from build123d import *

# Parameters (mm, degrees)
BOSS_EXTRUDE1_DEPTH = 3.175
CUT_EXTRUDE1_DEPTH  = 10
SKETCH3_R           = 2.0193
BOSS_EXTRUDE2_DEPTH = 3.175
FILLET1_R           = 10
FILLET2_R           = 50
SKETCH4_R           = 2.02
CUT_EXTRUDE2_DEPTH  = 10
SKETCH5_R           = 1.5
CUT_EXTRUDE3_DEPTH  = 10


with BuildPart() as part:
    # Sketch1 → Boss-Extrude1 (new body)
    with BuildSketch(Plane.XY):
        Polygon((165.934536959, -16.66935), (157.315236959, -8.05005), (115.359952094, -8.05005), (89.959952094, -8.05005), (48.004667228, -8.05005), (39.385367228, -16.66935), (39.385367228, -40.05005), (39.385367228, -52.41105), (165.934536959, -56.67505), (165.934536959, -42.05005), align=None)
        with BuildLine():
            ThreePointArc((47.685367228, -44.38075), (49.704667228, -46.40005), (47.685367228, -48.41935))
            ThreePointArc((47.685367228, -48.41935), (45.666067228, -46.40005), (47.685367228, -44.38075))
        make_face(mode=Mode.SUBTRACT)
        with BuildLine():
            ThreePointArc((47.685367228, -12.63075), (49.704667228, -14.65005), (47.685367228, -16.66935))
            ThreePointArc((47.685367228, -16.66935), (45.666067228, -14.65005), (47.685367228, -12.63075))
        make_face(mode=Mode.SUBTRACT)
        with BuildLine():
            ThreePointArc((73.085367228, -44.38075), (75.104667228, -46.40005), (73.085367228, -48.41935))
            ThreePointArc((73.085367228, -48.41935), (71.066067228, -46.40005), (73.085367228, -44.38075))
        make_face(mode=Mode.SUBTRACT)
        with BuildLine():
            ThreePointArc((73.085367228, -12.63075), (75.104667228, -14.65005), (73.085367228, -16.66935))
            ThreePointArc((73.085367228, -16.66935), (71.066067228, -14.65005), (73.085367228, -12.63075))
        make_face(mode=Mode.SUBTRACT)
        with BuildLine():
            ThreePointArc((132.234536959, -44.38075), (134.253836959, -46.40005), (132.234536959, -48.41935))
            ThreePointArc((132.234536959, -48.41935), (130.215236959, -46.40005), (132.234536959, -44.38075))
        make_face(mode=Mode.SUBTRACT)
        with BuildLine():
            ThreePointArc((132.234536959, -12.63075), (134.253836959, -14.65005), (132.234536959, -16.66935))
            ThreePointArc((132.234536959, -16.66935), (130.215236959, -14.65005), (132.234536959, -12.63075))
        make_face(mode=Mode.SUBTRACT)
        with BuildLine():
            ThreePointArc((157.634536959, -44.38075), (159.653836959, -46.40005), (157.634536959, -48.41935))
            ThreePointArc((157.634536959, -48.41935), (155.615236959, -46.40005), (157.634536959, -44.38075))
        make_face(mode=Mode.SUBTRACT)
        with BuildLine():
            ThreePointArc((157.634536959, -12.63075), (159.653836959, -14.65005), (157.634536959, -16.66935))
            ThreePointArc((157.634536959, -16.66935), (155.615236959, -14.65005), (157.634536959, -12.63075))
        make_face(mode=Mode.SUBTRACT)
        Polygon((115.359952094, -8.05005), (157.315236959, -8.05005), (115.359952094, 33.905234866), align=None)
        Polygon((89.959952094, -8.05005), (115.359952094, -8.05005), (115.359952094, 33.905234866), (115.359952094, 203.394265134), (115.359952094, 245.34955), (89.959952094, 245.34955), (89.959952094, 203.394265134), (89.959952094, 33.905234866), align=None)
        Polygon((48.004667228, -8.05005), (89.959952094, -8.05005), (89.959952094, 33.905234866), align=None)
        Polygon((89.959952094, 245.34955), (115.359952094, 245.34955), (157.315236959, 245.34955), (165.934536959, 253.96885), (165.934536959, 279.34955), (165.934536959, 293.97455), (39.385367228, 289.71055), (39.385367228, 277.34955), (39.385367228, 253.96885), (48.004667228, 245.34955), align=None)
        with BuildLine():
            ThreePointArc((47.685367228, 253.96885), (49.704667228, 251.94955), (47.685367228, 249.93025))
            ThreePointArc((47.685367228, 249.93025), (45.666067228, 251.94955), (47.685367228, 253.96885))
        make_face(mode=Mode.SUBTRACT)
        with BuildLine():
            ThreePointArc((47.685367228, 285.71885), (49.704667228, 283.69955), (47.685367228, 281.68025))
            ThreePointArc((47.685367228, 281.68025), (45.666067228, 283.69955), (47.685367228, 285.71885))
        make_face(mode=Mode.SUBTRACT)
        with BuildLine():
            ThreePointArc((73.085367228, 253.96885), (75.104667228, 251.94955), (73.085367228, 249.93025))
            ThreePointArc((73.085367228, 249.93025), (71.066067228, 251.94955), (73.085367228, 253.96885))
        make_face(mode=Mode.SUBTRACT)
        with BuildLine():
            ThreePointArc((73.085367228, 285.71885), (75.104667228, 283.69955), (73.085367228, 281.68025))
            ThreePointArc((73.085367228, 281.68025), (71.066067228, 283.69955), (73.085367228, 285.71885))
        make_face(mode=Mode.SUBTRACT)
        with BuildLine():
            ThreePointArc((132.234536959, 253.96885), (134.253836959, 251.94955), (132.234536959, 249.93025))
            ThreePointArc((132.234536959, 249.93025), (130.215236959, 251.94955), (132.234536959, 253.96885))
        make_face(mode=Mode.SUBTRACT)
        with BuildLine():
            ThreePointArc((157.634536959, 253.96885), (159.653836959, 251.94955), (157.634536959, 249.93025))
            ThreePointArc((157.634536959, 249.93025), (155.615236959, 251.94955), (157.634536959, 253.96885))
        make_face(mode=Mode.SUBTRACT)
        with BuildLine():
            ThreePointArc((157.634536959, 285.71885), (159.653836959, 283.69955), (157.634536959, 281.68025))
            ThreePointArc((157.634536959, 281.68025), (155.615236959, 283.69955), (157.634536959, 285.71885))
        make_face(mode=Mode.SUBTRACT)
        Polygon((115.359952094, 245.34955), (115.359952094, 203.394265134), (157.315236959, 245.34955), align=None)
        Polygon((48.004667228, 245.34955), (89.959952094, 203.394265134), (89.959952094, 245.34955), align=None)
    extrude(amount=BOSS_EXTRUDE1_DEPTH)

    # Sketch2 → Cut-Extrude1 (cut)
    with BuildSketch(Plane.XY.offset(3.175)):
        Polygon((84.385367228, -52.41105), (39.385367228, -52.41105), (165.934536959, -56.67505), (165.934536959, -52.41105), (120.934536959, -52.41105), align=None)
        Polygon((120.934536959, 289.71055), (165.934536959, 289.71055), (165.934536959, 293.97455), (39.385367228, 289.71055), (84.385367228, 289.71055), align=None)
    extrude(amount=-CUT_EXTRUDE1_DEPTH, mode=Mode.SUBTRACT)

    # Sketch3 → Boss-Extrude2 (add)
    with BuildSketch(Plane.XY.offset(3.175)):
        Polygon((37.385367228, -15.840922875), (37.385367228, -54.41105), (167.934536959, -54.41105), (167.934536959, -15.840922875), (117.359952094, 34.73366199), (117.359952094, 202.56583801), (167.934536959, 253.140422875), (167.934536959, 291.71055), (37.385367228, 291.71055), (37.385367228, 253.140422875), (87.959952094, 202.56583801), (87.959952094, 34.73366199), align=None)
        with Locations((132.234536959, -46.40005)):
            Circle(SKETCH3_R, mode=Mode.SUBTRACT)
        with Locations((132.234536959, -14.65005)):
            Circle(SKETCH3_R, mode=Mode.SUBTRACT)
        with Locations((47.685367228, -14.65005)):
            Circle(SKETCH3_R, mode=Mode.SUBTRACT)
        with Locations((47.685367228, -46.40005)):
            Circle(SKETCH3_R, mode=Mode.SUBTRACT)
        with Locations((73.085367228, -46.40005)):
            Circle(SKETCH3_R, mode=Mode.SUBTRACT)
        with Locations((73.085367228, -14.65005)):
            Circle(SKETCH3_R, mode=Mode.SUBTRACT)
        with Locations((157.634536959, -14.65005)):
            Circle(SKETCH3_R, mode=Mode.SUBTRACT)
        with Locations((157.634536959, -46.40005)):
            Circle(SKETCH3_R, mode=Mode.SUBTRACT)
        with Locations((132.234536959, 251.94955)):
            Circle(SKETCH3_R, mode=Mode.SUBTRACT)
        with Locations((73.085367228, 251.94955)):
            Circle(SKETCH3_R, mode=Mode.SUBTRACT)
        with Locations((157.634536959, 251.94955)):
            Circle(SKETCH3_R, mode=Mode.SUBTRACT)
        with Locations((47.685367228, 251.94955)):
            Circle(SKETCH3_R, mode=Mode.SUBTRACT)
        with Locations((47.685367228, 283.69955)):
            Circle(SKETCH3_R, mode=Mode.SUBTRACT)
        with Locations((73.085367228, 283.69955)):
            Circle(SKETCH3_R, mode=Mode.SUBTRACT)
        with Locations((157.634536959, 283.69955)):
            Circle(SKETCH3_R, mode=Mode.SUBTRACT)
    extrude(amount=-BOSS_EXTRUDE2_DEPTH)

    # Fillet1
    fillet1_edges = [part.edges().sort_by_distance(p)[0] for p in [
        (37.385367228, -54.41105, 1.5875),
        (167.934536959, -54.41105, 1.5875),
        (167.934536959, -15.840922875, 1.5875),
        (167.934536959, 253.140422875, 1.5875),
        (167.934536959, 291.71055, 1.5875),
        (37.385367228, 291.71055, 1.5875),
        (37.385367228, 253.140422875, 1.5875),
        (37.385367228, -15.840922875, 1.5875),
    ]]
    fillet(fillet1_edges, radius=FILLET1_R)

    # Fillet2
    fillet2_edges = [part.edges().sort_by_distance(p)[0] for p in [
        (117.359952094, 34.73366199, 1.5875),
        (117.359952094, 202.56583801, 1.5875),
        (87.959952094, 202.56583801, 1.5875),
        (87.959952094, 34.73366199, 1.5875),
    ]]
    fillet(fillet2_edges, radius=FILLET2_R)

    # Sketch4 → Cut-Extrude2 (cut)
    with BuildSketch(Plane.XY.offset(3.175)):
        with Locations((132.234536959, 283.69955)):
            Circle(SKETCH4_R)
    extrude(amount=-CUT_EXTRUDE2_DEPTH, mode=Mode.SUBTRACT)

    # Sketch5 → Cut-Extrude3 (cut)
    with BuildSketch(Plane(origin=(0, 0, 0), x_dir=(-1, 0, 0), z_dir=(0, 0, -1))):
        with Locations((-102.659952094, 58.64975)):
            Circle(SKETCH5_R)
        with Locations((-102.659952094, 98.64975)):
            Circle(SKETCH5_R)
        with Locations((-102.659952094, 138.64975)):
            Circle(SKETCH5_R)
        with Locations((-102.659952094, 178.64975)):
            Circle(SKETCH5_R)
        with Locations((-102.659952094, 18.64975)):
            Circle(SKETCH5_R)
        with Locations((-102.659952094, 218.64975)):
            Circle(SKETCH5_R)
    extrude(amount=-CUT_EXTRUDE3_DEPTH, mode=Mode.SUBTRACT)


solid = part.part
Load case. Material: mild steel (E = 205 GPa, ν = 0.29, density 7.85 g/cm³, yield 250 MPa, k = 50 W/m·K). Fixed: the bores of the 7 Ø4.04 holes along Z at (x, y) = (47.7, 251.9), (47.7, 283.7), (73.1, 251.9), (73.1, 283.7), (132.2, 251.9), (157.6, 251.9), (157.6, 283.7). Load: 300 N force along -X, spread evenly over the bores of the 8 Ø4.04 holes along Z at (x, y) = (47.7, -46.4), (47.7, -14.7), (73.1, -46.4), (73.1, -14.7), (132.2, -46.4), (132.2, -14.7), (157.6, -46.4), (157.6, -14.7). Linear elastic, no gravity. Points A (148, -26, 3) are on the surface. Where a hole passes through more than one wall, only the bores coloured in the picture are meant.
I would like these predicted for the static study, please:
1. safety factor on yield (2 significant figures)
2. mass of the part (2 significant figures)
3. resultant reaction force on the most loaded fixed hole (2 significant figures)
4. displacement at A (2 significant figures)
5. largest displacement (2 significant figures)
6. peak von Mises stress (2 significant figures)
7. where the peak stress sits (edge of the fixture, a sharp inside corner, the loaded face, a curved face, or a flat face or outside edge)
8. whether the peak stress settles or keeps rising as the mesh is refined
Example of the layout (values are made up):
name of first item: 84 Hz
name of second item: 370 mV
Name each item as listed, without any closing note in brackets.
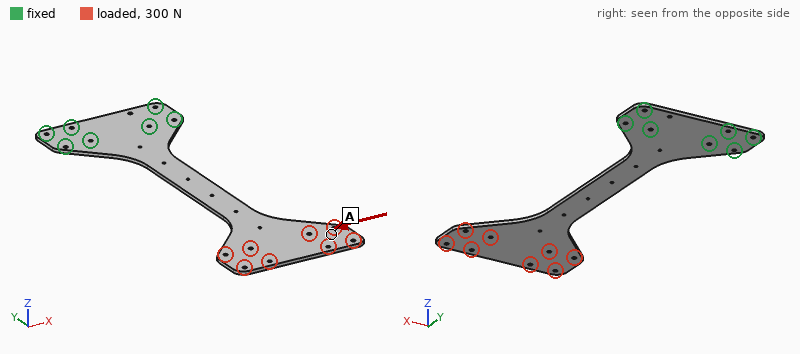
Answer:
safety factor on yield: 1.7
mass of the part: 570 g
resultant reaction force on the most loaded fixed hole: 770 N
displacement at A: 0.98 mm
largest displacement: 1.2 mm
peak von Mises stress: 150 MPa
where the peak stress sits: a curved face
whether the peak stress settles or keeps rising as the mesh is refined: settles
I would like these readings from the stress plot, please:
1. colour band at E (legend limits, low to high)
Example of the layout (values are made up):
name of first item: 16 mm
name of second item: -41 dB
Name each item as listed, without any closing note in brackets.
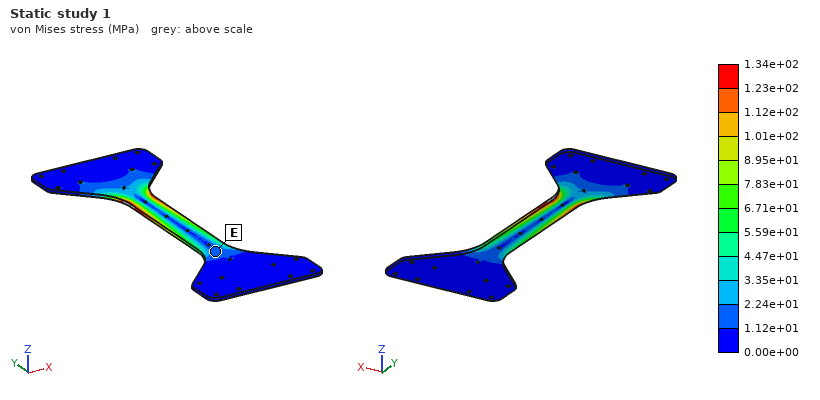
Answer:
colour band at E: 1.12e+01 to 2.24e+01 MPa
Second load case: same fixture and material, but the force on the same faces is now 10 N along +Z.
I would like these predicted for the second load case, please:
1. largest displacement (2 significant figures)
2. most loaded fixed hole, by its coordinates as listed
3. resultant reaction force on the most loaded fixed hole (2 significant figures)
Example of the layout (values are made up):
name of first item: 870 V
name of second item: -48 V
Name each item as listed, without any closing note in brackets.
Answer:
largest displacement: 4.0 mm
most loaded fixed hole, by its coordinates as listed: (73.1, 251.9)
resultant reaction force on the most loaded fixed hole: 31 N
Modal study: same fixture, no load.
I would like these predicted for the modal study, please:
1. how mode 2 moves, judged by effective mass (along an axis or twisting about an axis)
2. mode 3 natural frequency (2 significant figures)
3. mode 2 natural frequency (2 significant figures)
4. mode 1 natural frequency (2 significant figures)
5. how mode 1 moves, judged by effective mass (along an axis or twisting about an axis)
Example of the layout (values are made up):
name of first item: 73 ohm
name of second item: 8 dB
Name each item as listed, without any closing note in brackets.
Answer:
how mode 2 moves, judged by effective mass: twisting about Y
mode 3 natural frequency: 170 Hz
mode 2 natural frequency: 110 Hz
mode 1 natural frequency: 18 Hz
how mode 1 moves, judged by effective mass: along Z
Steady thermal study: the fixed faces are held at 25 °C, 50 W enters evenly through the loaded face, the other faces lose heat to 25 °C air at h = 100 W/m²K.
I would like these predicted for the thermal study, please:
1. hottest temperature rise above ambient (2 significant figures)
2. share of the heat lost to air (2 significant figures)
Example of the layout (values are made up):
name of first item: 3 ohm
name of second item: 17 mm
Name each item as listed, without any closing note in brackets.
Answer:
hottest temperature rise above ambient: 52 K
share of the heat lost to air: 100 %
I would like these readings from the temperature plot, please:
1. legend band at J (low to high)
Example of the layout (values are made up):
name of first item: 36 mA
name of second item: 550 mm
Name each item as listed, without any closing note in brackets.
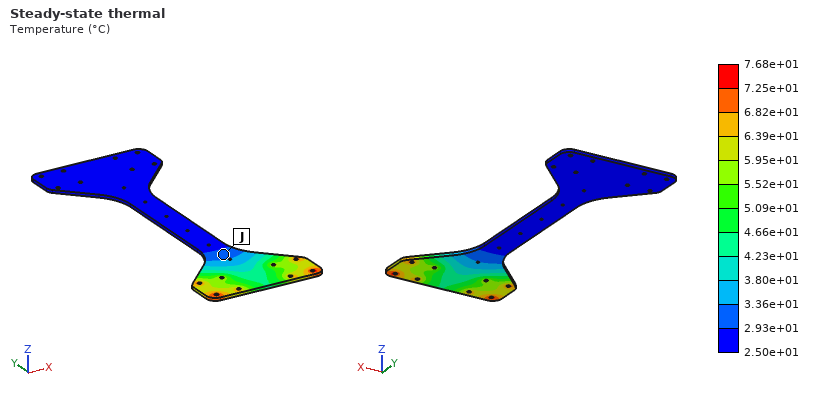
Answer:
legend band at J: 2.93e+01 to 3.36e+01 °C
